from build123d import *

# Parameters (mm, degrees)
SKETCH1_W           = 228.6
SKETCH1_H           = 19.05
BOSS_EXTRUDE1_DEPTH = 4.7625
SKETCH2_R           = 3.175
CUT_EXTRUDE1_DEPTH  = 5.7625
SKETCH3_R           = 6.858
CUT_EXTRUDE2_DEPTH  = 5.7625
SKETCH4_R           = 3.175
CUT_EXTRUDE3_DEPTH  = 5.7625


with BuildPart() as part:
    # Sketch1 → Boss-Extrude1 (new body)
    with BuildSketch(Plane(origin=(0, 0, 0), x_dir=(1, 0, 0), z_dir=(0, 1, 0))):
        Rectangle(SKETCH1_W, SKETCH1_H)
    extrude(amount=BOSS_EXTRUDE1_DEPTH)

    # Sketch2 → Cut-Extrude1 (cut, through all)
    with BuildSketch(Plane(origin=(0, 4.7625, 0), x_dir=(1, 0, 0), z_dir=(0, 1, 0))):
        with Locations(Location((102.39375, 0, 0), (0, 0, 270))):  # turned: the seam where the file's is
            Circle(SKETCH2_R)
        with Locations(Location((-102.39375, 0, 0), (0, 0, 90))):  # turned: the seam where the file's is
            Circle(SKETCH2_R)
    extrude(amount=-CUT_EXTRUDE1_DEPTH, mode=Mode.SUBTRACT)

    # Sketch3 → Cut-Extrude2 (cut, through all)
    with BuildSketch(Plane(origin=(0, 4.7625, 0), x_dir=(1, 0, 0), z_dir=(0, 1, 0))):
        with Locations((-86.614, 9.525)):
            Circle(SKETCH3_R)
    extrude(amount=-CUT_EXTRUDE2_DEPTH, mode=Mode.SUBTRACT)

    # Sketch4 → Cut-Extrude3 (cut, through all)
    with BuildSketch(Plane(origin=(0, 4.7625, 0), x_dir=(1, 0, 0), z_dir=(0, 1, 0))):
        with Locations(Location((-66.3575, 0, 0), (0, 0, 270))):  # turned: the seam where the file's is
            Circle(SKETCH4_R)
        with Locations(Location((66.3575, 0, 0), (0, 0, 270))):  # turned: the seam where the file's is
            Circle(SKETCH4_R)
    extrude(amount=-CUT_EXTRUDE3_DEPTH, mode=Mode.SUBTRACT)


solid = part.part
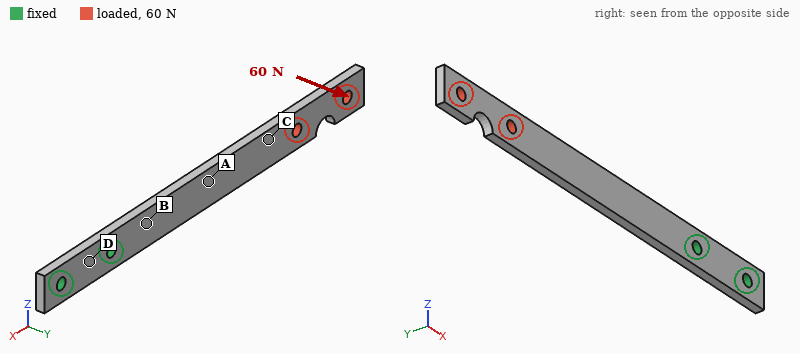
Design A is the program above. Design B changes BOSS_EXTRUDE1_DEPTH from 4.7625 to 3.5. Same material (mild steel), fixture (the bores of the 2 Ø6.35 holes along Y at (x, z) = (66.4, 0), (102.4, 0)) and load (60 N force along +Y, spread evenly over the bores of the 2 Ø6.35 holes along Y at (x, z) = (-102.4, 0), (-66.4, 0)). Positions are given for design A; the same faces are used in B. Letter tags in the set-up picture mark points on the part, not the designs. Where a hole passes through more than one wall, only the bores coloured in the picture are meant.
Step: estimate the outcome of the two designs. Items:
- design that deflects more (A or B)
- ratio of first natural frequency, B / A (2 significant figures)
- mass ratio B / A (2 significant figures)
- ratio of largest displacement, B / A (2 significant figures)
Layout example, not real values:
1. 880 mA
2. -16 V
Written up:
1. B
2. 0.74
3. 0.73
4. 2.5
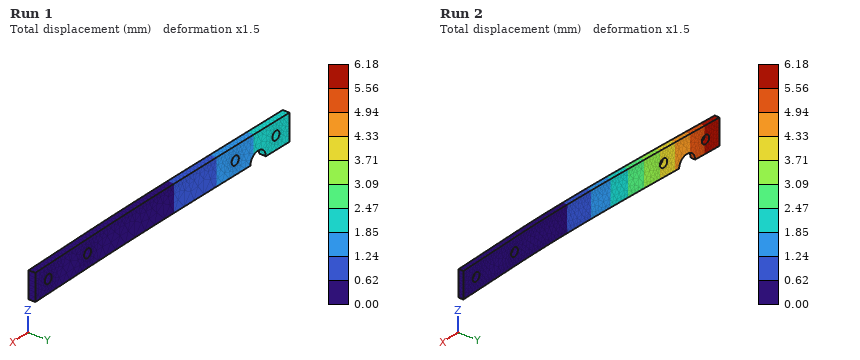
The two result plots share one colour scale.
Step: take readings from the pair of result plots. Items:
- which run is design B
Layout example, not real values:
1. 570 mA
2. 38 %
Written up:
1. Run 2
